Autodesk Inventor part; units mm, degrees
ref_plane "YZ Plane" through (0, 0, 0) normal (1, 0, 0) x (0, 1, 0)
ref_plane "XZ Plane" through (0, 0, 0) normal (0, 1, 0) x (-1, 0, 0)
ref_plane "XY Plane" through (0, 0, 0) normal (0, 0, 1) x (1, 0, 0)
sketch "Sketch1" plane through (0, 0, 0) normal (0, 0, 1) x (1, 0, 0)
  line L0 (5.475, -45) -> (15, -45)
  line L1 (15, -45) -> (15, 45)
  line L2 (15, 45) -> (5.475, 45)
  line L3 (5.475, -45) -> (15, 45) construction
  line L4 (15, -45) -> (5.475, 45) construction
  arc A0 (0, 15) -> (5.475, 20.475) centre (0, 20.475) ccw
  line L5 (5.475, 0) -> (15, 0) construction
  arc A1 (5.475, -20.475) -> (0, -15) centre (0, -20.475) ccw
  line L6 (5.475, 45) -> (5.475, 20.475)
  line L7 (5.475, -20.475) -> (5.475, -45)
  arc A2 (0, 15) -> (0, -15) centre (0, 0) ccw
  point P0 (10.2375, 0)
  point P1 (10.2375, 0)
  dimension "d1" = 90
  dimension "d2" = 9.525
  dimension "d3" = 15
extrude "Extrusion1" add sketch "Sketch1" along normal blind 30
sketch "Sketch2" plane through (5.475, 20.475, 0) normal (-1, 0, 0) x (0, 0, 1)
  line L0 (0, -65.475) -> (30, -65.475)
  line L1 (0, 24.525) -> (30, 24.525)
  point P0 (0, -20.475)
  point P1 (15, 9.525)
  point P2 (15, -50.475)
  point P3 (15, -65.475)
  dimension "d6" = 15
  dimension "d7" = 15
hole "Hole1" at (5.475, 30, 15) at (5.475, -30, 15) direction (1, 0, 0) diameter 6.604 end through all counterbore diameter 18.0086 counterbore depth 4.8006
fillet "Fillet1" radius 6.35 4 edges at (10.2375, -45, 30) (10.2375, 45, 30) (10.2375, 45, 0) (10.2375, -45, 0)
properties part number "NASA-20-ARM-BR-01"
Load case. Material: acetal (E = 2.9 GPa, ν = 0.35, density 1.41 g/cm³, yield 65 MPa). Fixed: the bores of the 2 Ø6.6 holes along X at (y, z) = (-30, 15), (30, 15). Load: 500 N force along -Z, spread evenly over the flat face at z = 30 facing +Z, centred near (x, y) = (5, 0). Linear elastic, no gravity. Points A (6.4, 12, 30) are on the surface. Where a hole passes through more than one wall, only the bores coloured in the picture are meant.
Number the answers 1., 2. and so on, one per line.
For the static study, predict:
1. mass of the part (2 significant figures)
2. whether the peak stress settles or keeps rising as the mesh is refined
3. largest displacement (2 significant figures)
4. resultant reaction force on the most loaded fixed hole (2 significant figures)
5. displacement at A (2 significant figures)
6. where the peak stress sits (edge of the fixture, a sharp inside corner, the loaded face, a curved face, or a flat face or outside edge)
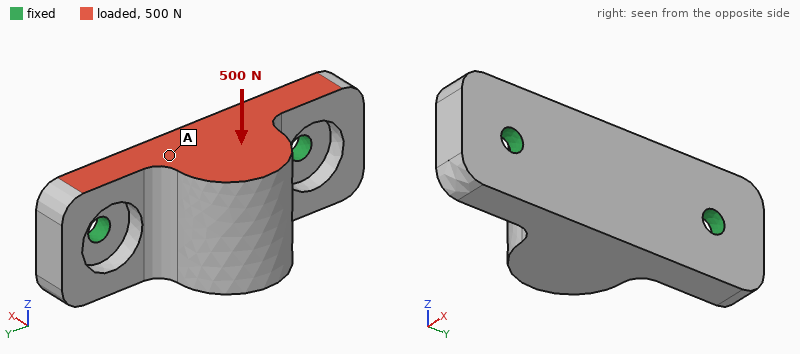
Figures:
1. 54 g
2. keeps rising
3. 0.29 mm
4. 250 N
5. 0.15 mm
6. edge of the fixture
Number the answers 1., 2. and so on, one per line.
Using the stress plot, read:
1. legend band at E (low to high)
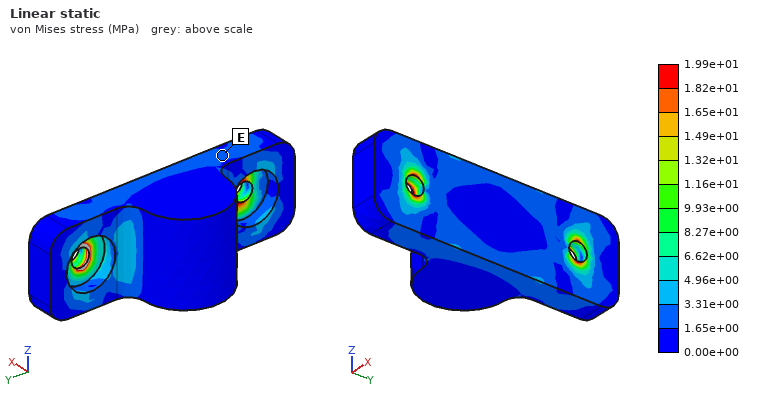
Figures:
1. 1.65e+00 to 3.31e+00 MPa
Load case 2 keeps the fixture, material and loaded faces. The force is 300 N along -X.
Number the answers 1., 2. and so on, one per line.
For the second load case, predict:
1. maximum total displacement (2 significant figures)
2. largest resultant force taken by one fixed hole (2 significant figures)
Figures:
1. 0.28 mm
2. 170 N
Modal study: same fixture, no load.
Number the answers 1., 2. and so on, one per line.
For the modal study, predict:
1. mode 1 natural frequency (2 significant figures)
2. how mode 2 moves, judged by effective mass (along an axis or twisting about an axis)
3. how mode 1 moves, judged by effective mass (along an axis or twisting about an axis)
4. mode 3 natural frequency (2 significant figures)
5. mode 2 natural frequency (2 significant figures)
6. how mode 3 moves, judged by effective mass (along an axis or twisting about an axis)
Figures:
1. 1100 Hz
2. along X
3. along Z
4. 3600 Hz
5. 2300 Hz
6. along Y
